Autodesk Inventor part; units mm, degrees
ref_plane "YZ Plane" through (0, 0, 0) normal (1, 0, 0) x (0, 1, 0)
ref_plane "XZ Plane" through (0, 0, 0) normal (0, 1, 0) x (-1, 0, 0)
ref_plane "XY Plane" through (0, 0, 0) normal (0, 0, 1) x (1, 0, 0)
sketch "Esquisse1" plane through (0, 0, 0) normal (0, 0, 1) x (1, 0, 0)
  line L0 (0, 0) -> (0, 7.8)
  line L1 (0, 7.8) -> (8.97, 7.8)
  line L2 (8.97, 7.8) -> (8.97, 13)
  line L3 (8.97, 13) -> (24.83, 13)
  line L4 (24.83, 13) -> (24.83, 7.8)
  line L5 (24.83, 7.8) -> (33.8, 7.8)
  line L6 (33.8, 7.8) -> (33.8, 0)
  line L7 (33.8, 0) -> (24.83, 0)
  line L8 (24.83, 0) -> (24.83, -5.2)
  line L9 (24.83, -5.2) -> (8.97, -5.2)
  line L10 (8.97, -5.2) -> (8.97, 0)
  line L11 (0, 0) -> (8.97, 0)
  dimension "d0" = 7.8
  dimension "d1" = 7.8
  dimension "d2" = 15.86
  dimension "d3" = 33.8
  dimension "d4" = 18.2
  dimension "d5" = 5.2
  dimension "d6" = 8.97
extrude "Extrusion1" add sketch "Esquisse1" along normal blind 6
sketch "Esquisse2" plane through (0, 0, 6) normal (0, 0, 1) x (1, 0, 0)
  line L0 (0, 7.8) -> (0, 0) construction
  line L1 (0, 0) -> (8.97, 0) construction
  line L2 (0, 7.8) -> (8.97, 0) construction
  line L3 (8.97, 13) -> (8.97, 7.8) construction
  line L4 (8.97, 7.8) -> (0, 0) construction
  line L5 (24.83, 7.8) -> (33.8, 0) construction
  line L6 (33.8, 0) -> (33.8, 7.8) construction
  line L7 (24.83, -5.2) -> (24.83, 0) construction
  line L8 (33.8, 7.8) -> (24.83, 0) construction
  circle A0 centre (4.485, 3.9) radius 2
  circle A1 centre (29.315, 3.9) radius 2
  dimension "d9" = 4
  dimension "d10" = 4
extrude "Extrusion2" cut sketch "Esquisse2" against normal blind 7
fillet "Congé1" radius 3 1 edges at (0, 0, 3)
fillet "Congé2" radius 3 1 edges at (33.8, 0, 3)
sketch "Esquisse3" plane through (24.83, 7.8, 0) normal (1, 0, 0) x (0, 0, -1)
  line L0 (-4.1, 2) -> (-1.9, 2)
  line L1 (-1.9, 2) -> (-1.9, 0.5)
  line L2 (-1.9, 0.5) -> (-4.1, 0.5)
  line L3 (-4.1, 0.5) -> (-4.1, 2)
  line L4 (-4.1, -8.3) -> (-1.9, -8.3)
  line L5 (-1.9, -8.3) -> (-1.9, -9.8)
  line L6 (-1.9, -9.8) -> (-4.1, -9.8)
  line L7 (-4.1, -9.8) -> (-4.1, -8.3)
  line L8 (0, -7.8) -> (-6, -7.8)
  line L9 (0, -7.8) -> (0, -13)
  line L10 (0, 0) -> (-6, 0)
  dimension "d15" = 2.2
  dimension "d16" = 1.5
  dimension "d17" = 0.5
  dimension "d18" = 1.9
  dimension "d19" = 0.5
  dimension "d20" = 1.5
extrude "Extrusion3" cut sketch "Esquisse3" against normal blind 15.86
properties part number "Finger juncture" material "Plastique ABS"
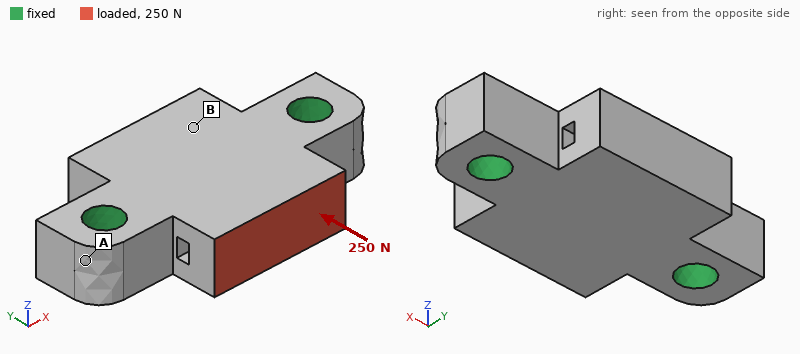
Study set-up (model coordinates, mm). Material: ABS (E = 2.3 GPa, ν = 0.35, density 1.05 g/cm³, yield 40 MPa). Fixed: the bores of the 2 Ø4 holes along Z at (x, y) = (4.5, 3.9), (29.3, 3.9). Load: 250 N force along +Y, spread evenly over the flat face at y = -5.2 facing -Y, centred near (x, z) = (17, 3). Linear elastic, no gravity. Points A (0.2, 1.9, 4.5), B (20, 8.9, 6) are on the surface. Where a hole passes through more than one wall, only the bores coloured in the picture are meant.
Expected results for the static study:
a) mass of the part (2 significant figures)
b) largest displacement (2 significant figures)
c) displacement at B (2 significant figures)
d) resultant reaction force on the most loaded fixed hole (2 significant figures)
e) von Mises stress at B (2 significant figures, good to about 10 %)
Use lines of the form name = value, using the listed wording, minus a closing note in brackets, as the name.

mass of the part = 2.4 g
largest displacement = 34 µm
displacement at B = 22 µm
resultant reaction force on the most loaded fixed hole = 130 N
von Mises stress at B = 2.3 MPa
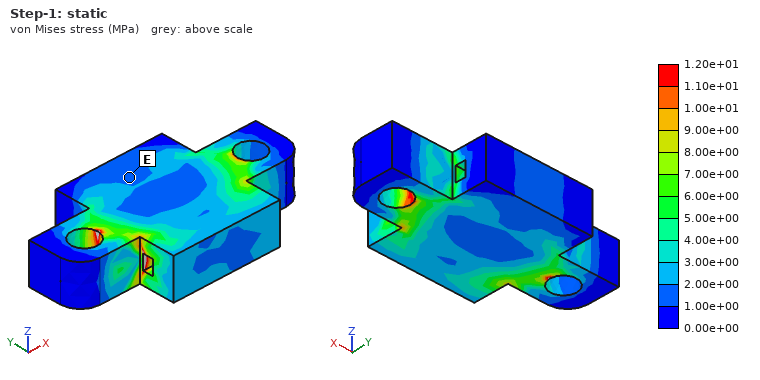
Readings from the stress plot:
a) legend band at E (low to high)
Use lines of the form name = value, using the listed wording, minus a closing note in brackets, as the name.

legend band at E = 1.00e+00 to 2.00e+00 MPa
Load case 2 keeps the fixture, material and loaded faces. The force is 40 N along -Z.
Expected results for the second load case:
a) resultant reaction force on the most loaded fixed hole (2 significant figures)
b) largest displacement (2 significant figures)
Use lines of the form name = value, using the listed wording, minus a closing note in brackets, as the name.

resultant reaction force on the most loaded fixed hole = 20 N
largest displacement = 56 µm
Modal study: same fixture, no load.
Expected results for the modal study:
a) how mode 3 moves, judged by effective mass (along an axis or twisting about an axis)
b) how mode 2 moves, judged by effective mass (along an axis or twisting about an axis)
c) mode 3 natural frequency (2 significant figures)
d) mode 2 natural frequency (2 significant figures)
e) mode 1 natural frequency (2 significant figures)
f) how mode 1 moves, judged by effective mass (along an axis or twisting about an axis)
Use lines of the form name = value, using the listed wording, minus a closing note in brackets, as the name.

how mode 3 moves, judged by effective mass = along Y
how mode 2 moves, judged by effective mass = along Z
mode 3 natural frequency = 12 kHz
mode 2 natural frequency = 8900 Hz
mode 1 natural frequency = 6900 Hz
how mode 1 moves, judged by effective mass = twisting about X
